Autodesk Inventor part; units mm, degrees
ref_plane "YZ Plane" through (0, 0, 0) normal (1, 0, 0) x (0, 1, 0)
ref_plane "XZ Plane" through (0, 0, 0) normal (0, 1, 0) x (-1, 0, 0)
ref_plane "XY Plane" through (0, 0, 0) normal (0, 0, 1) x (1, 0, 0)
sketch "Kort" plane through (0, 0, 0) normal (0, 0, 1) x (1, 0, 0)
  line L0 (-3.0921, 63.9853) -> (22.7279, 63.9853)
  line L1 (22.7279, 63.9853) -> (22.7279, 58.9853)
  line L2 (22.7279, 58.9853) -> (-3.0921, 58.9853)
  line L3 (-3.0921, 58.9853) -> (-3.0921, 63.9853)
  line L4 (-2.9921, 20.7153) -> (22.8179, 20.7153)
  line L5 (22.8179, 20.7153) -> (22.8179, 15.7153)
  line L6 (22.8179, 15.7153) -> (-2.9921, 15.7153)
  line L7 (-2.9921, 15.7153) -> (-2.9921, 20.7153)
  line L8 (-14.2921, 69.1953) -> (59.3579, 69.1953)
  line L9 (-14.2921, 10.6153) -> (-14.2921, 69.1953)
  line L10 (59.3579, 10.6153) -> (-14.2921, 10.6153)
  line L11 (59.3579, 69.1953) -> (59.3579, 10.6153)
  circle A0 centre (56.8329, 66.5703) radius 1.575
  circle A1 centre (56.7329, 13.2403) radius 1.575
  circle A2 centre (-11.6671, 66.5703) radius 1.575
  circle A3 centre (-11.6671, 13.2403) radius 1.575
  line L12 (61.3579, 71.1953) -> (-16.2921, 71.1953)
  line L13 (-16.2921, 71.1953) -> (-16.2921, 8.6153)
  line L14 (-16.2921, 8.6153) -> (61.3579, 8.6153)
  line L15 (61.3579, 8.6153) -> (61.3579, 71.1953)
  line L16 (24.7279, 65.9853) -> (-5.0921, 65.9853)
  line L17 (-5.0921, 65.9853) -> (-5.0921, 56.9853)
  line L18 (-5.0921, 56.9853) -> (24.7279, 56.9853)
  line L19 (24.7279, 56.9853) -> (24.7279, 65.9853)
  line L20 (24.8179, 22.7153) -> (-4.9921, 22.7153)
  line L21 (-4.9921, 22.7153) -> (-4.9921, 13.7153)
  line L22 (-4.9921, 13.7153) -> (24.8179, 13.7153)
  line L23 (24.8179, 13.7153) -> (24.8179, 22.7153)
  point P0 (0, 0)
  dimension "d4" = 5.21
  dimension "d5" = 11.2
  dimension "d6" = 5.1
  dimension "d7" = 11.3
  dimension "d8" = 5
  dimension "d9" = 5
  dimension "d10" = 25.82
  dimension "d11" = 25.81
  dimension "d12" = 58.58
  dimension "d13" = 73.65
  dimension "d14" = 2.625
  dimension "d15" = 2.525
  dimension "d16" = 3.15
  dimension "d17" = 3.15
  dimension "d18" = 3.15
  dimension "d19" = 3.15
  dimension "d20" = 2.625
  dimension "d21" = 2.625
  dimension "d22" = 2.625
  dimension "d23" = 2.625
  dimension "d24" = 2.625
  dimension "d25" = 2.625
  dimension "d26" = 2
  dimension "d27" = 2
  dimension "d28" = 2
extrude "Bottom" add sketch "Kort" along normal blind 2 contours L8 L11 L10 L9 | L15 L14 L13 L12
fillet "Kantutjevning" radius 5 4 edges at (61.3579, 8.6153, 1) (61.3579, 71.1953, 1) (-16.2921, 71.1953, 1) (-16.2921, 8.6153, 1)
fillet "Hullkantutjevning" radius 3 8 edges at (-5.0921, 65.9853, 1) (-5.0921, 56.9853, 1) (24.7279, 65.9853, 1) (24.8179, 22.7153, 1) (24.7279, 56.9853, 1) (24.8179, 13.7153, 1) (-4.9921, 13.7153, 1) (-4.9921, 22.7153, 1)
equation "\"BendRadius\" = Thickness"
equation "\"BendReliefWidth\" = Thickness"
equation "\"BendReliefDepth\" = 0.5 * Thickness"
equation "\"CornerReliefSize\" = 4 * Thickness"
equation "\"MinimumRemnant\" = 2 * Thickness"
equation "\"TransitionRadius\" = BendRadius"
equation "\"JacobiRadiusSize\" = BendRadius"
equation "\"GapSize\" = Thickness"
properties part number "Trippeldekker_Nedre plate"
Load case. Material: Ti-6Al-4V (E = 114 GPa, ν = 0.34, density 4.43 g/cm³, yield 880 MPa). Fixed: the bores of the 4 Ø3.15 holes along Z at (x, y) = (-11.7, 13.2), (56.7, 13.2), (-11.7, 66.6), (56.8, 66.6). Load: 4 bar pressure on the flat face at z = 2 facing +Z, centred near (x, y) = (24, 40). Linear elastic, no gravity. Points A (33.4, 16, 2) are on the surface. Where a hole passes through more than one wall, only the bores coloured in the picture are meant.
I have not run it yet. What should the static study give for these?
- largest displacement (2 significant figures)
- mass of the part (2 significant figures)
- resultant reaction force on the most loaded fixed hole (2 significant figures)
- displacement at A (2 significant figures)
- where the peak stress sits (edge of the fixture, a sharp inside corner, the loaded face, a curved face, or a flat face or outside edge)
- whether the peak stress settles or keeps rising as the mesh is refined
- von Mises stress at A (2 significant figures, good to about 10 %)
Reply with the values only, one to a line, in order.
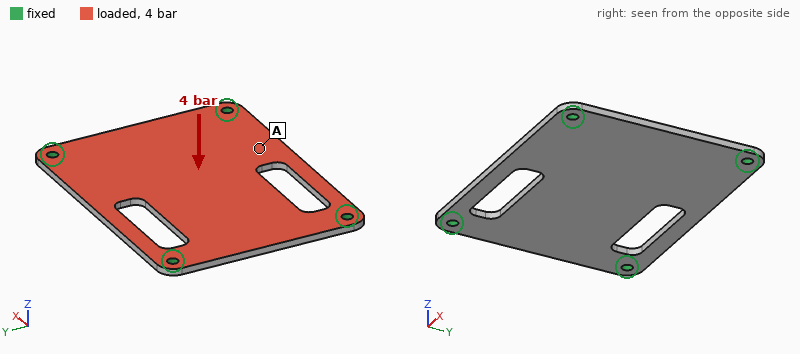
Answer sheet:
0.55 mm
38 g
460 N
0.36 mm
edge of the fixture
keeps rising
83 MPa
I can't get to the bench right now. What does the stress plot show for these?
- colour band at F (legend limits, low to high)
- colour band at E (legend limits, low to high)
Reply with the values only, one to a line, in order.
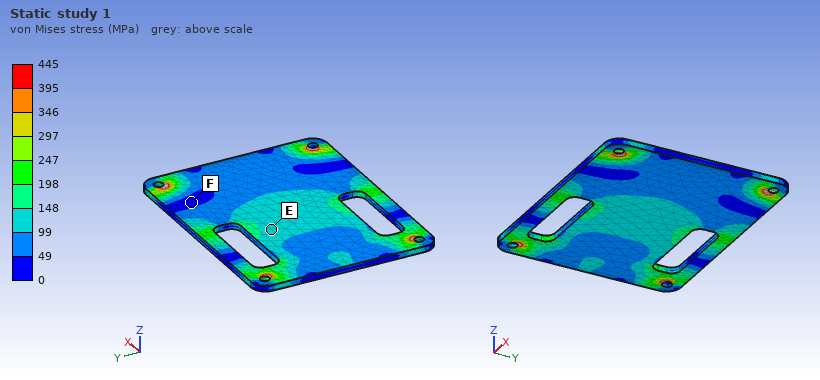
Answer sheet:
0 to 49 MPa
99 to 148 MPa
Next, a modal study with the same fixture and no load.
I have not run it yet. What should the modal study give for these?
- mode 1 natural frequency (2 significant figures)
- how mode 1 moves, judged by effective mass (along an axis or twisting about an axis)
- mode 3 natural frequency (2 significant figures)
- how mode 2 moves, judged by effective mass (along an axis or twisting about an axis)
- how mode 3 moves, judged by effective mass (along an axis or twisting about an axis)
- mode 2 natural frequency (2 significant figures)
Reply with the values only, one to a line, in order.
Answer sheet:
1700 Hz
along Z
3500 Hz
twisting about X
twisting about Y
2800 Hz
